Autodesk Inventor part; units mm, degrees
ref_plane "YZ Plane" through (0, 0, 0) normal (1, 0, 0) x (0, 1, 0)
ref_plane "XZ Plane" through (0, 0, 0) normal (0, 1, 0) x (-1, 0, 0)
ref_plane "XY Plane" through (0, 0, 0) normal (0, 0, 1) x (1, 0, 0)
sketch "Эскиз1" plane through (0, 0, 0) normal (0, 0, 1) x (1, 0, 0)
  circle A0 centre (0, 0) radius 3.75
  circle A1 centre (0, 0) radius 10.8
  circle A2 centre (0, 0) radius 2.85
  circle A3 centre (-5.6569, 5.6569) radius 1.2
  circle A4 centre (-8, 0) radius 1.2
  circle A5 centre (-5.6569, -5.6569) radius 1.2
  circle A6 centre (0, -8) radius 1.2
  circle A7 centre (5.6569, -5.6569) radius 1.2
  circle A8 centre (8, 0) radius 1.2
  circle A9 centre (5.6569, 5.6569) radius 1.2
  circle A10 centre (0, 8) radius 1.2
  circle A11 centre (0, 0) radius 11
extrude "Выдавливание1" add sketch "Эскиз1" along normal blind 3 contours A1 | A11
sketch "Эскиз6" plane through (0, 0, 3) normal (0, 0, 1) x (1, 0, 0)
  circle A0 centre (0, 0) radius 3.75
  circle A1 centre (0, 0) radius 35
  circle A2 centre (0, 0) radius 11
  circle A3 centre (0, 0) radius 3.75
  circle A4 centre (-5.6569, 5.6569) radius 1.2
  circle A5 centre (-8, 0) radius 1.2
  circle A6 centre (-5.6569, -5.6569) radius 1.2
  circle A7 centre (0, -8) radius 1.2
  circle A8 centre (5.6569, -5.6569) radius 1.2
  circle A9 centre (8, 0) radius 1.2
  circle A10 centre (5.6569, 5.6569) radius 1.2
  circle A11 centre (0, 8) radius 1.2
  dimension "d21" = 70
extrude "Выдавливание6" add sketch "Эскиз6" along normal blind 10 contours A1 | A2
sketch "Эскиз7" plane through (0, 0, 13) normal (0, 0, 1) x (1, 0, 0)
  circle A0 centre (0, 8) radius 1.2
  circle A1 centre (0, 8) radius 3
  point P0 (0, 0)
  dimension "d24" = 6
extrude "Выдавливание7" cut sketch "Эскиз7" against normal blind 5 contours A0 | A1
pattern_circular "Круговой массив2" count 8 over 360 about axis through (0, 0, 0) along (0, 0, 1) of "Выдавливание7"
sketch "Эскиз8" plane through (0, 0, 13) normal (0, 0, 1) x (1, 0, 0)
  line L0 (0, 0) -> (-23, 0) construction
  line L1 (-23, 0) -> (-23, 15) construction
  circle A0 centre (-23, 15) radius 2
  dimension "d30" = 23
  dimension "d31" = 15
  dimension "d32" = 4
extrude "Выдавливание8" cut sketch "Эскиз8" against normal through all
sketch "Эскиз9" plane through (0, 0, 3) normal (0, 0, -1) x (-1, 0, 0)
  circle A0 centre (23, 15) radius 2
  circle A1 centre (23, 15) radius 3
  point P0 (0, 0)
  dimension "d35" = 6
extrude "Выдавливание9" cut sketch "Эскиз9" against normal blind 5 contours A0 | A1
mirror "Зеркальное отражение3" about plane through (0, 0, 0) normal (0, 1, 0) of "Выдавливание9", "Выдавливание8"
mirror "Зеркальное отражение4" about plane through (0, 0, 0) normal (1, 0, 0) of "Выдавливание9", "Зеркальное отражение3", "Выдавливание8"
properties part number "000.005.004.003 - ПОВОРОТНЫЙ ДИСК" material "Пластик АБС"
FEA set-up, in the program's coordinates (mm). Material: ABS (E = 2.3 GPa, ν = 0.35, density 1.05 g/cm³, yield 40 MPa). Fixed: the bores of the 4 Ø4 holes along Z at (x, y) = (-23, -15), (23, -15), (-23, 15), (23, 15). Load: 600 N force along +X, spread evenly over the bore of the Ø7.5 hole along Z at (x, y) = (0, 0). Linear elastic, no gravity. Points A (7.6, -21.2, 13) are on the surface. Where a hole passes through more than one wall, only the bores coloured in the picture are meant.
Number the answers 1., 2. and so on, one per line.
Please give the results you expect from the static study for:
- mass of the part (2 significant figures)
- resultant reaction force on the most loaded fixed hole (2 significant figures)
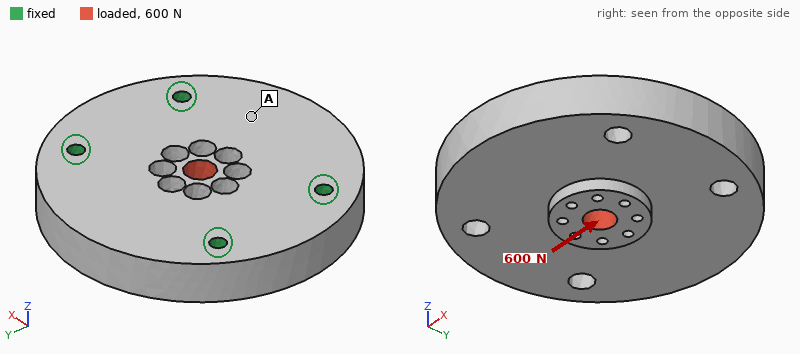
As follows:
1. 39 g
2. 160 N
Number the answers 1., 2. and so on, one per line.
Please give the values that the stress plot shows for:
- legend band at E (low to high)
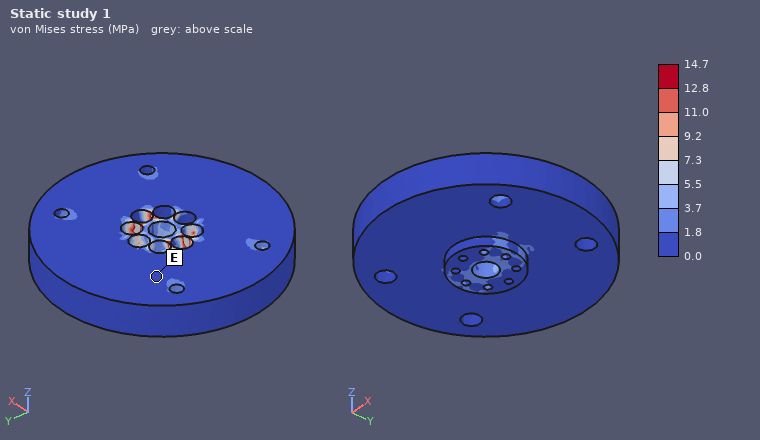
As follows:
1. 0.0 to 1.8 MPa
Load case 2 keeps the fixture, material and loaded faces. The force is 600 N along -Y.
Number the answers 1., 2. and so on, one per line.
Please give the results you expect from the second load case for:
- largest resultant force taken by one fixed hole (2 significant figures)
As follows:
1. 160 N
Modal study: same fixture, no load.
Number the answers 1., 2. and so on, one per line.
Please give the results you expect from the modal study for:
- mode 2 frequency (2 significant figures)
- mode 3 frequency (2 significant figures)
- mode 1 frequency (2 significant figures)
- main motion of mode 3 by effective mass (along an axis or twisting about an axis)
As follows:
1. 3200 Hz
2. 5100 Hz
3. 3100 Hz
4. along Z
